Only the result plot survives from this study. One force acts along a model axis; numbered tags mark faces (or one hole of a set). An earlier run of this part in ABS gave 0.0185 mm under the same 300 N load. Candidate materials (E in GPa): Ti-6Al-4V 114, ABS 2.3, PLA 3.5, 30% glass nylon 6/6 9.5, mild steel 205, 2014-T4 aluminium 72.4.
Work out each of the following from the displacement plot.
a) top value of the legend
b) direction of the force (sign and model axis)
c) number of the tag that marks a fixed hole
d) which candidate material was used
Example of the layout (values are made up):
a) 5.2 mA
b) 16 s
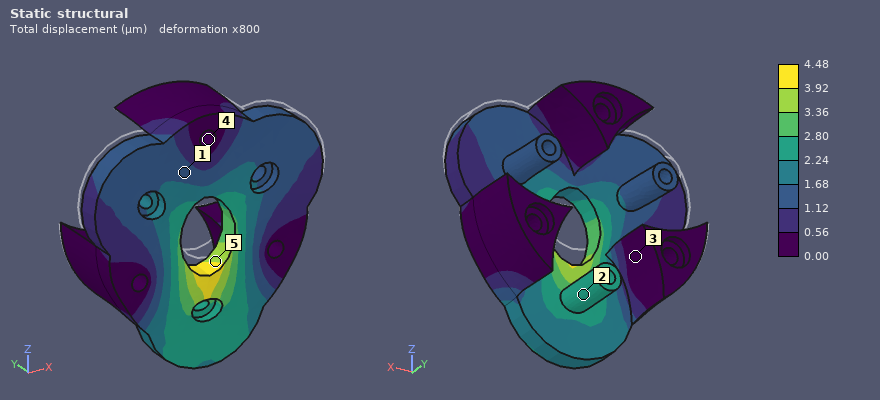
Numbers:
a) 4.48 µm
b) -Z
c) 4
d) 30% glass nylon 6/6
